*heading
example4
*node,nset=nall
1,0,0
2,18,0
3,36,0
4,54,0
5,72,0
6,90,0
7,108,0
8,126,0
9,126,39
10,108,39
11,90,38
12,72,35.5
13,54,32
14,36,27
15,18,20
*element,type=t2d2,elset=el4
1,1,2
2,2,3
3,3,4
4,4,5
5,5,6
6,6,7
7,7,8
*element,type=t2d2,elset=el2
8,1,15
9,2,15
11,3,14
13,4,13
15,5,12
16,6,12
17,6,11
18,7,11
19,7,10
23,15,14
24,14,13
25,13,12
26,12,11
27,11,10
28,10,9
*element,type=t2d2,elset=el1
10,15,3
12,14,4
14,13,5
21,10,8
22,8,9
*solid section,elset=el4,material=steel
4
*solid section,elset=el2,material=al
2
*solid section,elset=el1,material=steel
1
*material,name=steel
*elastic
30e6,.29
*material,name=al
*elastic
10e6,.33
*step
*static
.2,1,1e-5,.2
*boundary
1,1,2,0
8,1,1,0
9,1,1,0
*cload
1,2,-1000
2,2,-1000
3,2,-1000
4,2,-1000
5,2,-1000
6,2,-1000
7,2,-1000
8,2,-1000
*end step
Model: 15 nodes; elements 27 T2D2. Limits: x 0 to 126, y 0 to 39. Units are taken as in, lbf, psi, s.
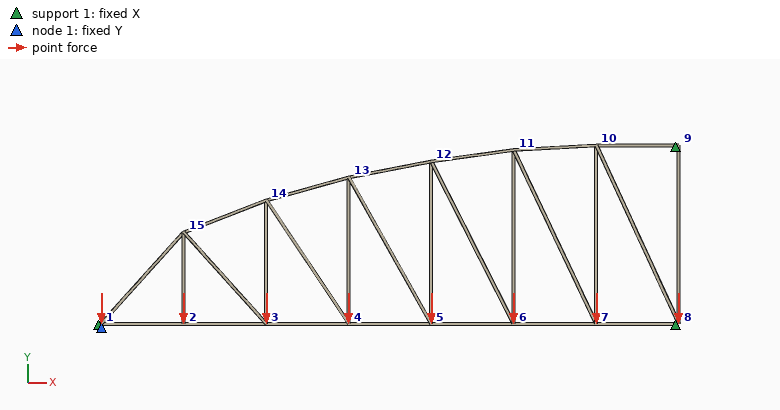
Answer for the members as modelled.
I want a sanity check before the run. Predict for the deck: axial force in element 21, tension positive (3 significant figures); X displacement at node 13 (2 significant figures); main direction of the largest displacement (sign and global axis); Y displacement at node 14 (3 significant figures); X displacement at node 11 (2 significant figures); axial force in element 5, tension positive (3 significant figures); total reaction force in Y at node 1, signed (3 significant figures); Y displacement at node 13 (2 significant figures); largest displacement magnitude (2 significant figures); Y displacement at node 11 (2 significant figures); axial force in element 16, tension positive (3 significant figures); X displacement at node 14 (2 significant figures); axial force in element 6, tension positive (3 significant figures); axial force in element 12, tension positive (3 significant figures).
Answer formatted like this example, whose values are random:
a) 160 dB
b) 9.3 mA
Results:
a) 1100 lbf
b) 0.036 in
c) -Y
d) -0.0835 in
e) 0.022 in
f) 1600 lbf
g) 8000 lbf
h) -0.11 in
i) 0.18 in
j) -0.16 in
k) 1520 lbf
l) 0.038 in
m) 2290 lbf
n) 2630 lbf
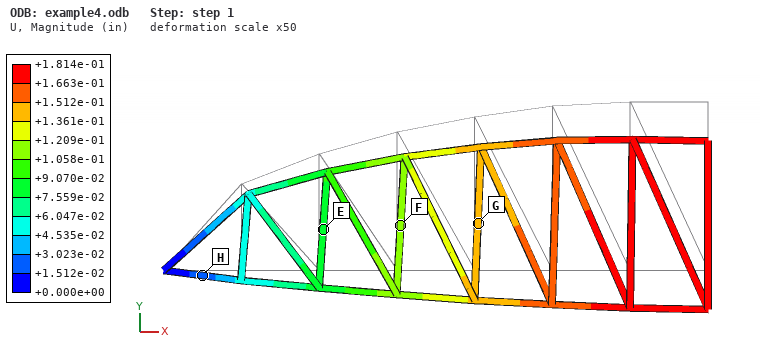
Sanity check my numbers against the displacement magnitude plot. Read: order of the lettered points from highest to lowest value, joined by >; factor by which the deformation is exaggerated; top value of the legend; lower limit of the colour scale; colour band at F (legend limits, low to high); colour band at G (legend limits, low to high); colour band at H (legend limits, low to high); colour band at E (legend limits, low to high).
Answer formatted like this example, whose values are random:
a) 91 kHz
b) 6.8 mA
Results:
a) G > F > E > H
b) 50
c) +1.814e-01 in
d) +0.000e+00 in
e) +1.058e-01 to +1.209e-01 in
f) +1.361e-01 to +1.512e-01 in
g) +1.512e-02 to +3.023e-02 in
h) +7.559e-02 to +9.070e-02 in
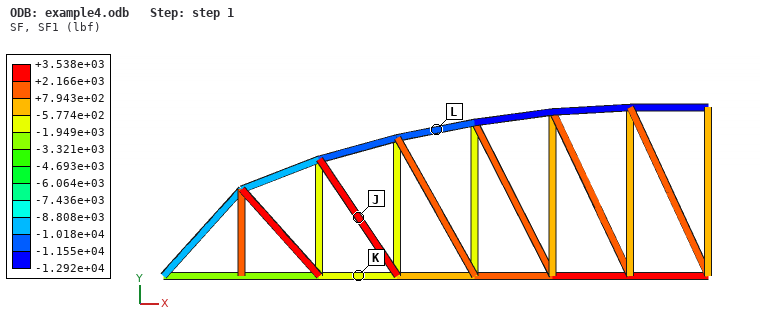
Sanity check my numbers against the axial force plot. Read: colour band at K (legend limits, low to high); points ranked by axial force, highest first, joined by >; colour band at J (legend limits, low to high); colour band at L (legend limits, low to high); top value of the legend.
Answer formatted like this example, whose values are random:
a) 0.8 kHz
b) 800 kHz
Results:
a) -1.949e+03 to -5.774e+02 lbf
b) J > K > L
c) +2.166e+03 to +3.538e+03 lbf
d) -1.155e+04 to -1.018e+04 lbf
e) +3.538e+03 lbf
